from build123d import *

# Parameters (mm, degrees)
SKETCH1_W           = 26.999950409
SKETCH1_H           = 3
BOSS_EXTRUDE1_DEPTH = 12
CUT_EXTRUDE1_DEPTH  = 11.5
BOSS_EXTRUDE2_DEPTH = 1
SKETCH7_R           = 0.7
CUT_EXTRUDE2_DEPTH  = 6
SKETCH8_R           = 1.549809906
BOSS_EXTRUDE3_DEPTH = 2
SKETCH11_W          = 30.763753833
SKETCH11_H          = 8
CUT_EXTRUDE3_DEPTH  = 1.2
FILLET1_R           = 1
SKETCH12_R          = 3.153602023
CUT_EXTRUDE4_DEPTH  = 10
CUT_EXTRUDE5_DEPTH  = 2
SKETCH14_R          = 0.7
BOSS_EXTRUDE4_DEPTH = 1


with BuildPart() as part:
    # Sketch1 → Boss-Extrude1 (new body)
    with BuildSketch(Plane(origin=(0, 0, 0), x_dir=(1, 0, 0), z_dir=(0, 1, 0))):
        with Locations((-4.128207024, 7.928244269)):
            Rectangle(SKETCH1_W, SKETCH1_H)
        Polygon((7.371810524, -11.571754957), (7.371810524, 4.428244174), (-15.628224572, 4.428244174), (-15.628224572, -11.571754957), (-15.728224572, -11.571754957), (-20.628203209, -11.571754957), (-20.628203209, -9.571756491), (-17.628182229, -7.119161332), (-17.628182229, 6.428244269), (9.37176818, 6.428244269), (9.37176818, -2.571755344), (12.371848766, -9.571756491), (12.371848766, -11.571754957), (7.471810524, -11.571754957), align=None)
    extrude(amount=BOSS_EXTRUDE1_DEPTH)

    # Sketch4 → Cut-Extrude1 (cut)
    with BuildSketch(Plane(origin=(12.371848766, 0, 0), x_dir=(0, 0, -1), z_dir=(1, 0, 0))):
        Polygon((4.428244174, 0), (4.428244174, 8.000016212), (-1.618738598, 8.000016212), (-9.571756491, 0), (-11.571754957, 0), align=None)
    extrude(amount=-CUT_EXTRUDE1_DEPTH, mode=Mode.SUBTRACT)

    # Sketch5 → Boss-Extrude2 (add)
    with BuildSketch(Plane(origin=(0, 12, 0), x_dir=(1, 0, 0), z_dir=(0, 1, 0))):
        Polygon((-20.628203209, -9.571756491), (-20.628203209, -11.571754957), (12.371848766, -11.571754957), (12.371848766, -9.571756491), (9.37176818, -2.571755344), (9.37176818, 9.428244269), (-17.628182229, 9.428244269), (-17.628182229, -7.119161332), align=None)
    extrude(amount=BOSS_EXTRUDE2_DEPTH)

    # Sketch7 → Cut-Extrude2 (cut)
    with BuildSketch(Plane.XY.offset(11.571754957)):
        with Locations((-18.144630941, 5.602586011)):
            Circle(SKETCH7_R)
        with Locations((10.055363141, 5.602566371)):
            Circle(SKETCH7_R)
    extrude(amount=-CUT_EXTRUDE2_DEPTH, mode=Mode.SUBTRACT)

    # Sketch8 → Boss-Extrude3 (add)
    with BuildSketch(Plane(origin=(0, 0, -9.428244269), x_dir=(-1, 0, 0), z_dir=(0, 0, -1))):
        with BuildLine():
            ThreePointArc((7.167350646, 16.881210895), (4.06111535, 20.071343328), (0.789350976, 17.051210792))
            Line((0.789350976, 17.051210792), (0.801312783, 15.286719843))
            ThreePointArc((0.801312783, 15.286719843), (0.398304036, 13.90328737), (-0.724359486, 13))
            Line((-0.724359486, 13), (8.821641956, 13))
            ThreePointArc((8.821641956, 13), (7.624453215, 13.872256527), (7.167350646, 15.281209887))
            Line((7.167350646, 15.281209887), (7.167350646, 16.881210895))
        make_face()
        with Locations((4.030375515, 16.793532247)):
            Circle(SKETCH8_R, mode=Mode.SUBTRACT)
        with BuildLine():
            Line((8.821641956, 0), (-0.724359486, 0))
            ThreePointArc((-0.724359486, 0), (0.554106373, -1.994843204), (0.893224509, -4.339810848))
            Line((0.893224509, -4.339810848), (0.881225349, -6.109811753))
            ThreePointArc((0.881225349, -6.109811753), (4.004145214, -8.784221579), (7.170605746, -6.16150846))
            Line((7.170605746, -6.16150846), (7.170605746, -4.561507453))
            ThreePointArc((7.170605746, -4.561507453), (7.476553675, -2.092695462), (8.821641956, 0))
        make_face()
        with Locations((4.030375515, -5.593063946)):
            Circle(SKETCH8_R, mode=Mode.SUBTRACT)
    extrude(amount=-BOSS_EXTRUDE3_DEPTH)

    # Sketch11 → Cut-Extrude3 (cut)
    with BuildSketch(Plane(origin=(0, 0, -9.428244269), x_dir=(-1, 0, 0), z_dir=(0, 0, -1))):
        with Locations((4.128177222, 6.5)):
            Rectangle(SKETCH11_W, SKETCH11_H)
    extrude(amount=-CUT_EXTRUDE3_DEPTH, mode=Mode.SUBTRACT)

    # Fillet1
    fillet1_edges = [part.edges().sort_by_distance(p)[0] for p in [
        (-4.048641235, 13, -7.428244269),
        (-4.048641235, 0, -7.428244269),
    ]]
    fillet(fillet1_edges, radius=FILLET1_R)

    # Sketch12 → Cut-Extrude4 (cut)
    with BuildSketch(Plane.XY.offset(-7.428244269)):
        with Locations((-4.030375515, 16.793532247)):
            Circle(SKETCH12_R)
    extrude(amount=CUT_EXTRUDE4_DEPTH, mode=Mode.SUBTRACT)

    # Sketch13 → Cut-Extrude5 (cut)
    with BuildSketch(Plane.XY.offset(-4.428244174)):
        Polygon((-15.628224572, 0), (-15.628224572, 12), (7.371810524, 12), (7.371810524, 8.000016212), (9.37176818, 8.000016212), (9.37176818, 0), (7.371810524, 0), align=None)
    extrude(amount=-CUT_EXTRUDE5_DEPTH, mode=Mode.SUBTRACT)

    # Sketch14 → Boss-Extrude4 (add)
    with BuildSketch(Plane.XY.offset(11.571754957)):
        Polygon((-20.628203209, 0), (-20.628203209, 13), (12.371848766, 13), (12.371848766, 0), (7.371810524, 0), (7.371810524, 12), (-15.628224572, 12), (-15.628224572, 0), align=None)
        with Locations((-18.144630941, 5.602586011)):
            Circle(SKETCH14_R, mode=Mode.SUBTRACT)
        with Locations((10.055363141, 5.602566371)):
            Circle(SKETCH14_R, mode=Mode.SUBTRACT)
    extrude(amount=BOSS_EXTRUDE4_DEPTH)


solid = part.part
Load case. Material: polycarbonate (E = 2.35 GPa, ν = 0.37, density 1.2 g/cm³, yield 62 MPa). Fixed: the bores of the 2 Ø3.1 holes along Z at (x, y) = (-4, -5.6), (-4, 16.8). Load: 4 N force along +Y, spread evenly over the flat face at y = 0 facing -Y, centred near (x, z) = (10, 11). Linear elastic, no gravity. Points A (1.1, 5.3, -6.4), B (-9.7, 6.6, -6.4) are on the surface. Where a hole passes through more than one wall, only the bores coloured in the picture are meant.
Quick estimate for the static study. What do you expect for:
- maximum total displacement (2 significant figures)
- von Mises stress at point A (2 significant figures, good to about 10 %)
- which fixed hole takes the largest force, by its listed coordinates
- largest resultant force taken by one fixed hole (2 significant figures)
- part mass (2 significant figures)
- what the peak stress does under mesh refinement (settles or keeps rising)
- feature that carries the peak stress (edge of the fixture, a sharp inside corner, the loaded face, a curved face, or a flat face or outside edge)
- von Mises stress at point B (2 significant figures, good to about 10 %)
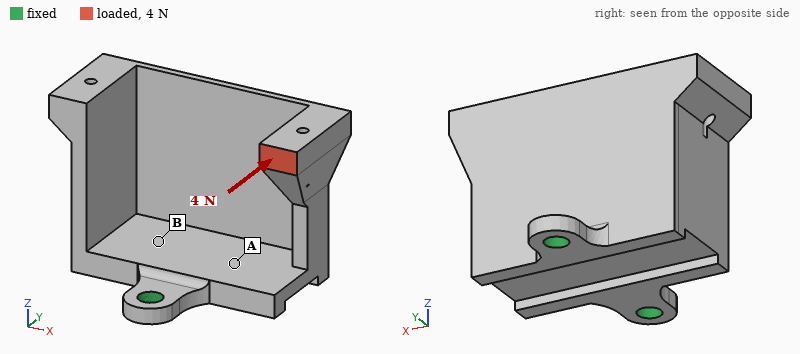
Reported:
0.54 mm
2.9 MPa
(-4, -5.6)
10 N
3.1 g
keeps rising
a sharp inside corner
0.84 MPa
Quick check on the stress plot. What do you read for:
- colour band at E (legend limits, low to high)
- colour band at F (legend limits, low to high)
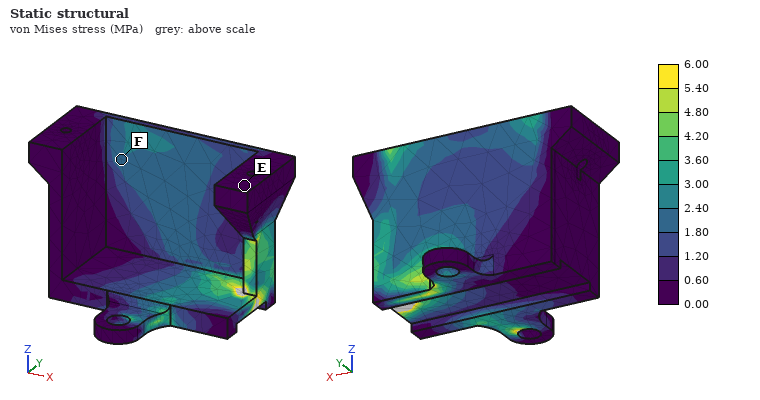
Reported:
0.00 to 0.60 MPa
1.80 to 2.40 MPa
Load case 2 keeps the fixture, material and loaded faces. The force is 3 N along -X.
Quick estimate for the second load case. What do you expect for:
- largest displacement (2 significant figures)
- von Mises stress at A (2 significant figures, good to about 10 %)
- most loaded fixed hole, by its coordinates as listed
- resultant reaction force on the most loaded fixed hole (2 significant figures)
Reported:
0.53 mm
0.80 MPa
(-4, -5.6)
2.5 N
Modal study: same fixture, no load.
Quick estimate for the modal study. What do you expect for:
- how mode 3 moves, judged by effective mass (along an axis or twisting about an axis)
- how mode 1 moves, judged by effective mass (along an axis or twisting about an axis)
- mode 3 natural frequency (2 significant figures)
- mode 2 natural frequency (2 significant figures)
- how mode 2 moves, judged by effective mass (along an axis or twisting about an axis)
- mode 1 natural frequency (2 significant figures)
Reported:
along Y
along X
940 Hz
690 Hz
along Y
530 Hz
